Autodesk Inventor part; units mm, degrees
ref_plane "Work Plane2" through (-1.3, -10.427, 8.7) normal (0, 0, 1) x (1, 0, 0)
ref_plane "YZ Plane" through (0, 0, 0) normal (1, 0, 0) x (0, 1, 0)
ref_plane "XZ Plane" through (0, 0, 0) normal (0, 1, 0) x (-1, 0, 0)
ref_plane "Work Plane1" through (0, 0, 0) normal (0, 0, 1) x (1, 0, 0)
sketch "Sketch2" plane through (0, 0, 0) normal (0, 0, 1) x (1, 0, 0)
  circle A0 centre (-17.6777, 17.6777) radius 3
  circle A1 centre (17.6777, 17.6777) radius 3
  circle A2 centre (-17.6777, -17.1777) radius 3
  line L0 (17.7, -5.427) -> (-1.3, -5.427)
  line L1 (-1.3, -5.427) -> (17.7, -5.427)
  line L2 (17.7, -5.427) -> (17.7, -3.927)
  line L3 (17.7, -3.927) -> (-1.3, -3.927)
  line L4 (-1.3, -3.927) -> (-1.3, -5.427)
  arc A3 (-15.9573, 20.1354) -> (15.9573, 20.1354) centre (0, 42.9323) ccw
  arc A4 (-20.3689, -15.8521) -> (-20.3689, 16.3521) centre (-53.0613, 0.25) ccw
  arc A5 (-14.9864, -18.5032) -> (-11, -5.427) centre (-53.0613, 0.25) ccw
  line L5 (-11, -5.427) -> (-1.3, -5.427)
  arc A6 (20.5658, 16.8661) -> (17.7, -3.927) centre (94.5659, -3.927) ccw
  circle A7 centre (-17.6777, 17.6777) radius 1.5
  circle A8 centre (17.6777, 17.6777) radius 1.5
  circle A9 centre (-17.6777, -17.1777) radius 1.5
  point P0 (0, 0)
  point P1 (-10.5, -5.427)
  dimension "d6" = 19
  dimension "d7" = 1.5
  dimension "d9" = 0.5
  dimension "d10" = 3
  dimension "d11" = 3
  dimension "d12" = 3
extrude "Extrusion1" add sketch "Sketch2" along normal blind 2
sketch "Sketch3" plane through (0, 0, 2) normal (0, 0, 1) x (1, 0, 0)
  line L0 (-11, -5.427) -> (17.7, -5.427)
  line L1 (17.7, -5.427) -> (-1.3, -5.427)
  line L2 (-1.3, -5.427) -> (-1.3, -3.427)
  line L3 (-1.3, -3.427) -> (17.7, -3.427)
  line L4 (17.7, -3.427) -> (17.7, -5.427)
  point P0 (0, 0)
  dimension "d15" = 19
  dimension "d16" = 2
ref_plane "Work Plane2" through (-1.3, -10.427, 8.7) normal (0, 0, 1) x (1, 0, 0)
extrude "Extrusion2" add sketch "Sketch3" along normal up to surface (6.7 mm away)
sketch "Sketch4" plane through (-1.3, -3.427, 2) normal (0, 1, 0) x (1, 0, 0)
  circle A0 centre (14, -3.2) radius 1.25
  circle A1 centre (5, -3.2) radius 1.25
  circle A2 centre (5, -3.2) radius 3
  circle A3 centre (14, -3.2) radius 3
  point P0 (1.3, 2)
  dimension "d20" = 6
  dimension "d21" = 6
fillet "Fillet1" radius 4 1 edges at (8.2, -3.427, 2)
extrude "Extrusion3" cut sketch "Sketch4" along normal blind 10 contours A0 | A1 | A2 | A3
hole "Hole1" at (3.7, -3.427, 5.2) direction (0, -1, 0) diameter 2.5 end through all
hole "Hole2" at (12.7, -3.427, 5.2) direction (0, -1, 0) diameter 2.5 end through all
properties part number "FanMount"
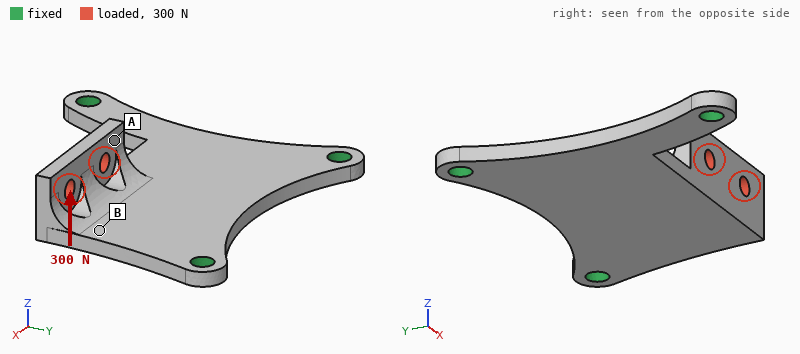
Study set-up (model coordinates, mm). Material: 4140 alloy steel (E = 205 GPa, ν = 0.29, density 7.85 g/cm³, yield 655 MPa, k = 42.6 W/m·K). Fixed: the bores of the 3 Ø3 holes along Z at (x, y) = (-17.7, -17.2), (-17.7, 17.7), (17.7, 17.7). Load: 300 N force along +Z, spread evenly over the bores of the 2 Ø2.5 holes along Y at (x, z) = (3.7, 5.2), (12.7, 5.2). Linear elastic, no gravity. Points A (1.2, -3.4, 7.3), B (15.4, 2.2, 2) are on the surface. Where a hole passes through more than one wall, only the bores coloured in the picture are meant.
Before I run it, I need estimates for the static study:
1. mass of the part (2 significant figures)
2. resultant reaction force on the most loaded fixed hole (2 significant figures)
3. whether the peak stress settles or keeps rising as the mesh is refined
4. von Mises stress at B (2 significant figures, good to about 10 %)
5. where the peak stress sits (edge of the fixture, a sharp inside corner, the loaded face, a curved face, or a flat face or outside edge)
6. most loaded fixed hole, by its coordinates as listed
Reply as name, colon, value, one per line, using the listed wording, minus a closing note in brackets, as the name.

mass of the part: 16 g
resultant reaction force on the most loaded fixed hole: 200 N
whether the peak stress settles or keeps rising as the mesh is refined: keeps rising
von Mises stress at B: 140 MPa
where the peak stress sits: edge of the fixture
most loaded fixed hole, by its coordinates as listed: (17.7, 17.7)
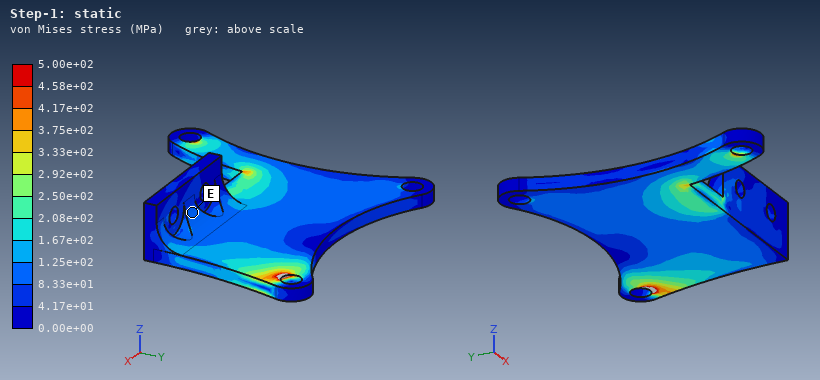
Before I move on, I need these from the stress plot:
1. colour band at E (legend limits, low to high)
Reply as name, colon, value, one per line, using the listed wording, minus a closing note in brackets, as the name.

colour band at E: 8.33e+01 to 1.25e+02 MPa
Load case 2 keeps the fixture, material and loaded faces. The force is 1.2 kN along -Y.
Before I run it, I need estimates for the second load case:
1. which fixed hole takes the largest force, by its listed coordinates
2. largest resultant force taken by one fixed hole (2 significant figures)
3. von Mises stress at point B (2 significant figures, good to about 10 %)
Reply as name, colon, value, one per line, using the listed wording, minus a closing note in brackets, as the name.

which fixed hole takes the largest force, by its listed coordinates: (17.7, 17.7)
largest resultant force taken by one fixed hole: 870 N
von Mises stress at point B: 260 MPa
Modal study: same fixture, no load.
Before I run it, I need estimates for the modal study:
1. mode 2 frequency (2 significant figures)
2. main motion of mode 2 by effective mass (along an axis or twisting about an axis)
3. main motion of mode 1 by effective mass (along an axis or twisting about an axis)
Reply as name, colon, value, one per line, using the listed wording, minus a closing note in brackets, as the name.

mode 2 frequency: 6600 Hz
main motion of mode 2 by effective mass: along Z
main motion of mode 1 by effective mass: along Z
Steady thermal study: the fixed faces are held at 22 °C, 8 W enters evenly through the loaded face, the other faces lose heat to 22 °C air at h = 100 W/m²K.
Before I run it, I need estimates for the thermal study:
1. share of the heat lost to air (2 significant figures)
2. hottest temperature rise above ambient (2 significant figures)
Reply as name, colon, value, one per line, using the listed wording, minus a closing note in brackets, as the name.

share of the heat lost to air: 63 %
hottest temperature rise above ambient: 66 K
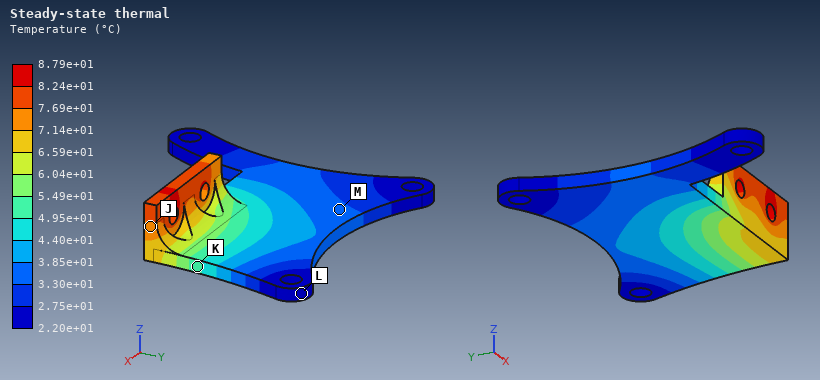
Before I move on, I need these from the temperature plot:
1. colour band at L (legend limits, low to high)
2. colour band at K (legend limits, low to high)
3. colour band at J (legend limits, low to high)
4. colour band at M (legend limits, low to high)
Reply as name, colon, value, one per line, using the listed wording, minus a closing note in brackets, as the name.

colour band at L: 2.20e+01 to 2.75e+01 °C
colour band at K: 4.95e+01 to 5.49e+01 °C
colour band at J: 7.14e+01 to 7.69e+01 °C
colour band at M: 3.30e+01 to 3.85e+01 °C
